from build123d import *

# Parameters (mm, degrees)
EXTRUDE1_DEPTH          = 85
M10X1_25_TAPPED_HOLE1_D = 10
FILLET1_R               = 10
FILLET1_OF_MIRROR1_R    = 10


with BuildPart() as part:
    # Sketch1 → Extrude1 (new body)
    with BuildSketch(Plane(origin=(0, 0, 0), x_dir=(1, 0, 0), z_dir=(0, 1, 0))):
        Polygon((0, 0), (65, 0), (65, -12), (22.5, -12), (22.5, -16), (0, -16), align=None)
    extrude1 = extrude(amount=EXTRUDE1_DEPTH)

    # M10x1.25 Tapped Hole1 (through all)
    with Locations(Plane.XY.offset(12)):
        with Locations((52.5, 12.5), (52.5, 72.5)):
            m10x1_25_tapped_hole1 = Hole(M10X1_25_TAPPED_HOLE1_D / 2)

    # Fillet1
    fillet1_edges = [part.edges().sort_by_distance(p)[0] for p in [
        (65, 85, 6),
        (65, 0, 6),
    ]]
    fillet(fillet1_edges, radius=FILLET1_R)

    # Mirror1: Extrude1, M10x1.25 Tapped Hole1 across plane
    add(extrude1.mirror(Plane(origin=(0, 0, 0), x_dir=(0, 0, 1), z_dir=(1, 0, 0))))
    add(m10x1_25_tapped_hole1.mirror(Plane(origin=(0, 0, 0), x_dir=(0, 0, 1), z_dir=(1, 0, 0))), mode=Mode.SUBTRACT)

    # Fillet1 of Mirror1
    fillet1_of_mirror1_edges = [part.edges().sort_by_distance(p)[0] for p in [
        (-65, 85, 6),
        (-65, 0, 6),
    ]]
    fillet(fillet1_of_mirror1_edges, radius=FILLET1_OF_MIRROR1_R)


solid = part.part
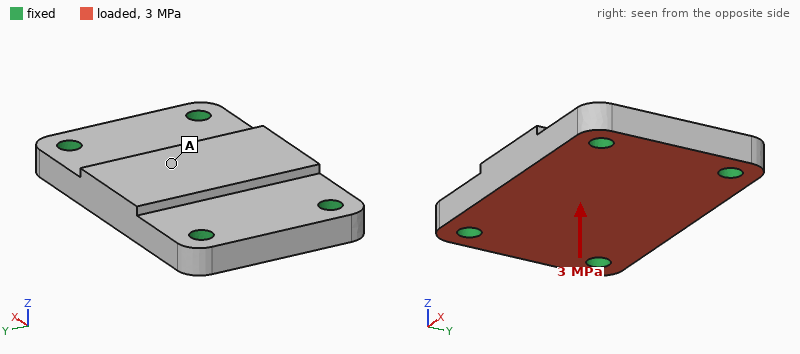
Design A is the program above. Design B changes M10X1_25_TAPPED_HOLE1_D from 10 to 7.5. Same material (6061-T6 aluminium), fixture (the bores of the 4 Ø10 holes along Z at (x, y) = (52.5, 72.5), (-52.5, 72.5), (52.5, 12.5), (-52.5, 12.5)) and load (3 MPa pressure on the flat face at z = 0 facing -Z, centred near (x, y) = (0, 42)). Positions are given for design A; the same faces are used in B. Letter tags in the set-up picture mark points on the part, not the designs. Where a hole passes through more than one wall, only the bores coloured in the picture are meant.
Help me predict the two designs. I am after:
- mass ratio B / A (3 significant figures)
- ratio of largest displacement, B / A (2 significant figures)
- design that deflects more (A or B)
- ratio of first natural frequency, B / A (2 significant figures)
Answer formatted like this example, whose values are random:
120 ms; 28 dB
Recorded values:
1.01; 1.1; B; 0.94
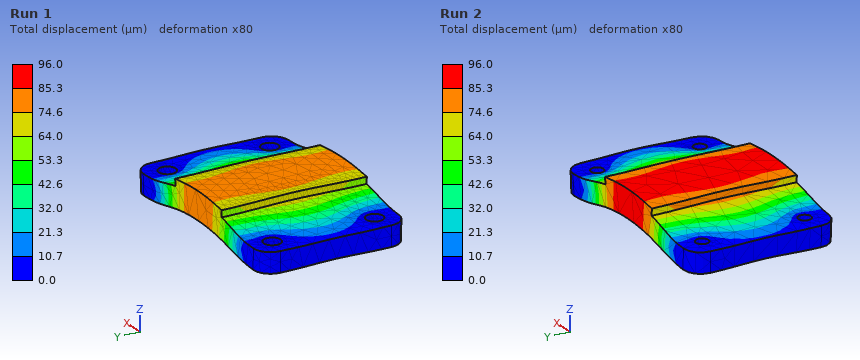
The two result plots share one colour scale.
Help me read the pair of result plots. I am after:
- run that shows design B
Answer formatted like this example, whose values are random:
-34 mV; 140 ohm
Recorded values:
Run 2
